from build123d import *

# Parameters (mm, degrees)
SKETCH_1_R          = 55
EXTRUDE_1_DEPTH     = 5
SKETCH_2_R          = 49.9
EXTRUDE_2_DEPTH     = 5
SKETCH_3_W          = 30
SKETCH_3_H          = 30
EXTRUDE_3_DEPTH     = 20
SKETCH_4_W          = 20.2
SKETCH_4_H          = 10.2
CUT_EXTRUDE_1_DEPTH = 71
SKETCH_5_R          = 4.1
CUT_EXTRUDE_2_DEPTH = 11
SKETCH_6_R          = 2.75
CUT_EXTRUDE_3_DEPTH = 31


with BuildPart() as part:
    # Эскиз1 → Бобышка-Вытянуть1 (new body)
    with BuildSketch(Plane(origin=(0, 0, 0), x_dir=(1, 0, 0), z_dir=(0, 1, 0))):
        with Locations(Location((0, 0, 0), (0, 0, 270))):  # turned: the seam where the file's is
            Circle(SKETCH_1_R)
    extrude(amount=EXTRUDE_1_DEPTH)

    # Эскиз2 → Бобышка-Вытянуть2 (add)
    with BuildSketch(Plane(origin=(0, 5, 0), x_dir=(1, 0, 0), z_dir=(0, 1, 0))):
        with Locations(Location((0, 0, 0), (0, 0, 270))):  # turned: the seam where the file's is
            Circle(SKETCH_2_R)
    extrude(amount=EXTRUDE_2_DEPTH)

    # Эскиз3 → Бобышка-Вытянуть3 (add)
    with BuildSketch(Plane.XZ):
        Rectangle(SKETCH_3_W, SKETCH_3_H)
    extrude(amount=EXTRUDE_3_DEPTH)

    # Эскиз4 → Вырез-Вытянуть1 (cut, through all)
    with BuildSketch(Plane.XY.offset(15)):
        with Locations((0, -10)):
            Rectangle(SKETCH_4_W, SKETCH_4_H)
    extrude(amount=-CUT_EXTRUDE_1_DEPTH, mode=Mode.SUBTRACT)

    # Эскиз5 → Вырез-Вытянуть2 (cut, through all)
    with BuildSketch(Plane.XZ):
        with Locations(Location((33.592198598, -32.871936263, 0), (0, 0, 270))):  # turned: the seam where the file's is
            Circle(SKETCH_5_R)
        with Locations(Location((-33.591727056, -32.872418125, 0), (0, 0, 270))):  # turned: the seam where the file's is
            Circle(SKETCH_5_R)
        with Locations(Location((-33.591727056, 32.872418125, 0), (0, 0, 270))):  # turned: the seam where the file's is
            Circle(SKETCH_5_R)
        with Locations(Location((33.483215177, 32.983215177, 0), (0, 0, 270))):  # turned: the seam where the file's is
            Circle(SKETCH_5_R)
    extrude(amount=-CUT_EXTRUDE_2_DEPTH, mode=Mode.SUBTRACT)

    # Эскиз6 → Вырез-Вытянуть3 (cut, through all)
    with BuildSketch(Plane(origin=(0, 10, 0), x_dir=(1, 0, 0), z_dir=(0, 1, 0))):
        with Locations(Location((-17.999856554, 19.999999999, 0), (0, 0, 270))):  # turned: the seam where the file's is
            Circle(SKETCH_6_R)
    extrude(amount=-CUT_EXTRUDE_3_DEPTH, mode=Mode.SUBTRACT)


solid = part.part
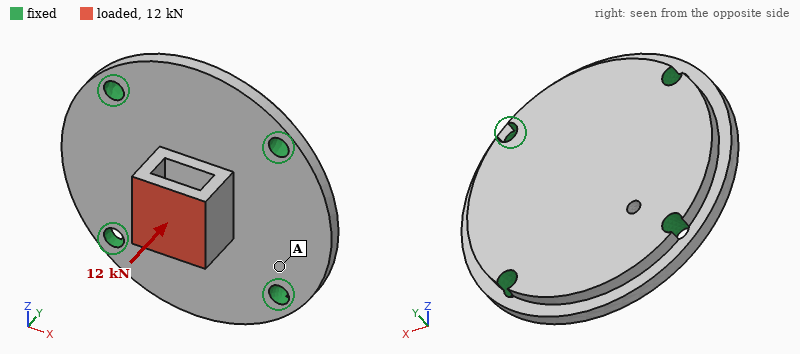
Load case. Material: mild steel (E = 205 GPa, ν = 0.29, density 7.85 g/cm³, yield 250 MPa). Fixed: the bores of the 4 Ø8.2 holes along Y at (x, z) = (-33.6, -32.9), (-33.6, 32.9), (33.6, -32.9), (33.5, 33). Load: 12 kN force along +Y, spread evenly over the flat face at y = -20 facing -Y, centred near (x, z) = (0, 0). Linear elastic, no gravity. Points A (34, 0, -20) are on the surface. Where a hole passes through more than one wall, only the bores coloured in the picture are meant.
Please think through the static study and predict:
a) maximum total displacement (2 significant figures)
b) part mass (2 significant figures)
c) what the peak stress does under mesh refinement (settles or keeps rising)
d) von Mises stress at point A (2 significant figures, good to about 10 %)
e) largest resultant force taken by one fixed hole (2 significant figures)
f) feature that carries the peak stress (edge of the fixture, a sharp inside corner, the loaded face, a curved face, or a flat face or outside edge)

34 µm
760 g
keeps rising
25 MPa
3.1 kN
edge of the fixture
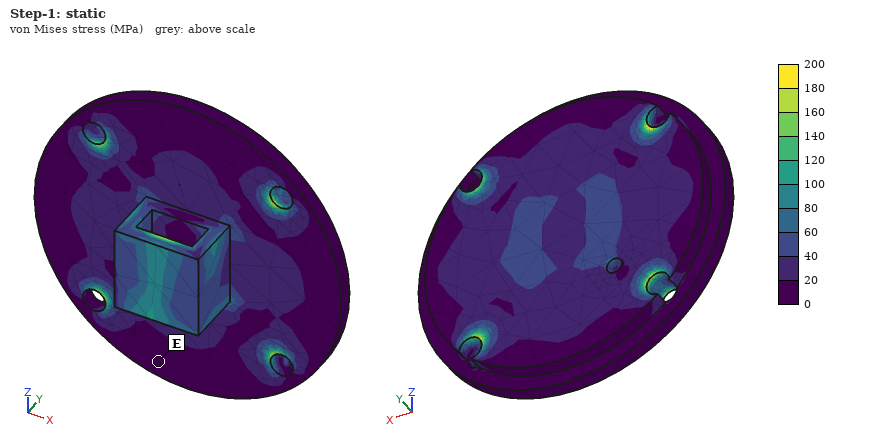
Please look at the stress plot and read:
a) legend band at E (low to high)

0 to 20 MPa
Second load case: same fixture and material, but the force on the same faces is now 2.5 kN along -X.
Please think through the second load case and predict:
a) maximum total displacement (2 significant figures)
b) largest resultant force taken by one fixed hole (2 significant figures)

15 µm
880 N
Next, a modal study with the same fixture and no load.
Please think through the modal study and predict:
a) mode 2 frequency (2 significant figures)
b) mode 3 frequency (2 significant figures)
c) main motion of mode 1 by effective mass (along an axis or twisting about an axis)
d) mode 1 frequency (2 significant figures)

9100 Hz
9100 Hz
along Y
7100 Hz
